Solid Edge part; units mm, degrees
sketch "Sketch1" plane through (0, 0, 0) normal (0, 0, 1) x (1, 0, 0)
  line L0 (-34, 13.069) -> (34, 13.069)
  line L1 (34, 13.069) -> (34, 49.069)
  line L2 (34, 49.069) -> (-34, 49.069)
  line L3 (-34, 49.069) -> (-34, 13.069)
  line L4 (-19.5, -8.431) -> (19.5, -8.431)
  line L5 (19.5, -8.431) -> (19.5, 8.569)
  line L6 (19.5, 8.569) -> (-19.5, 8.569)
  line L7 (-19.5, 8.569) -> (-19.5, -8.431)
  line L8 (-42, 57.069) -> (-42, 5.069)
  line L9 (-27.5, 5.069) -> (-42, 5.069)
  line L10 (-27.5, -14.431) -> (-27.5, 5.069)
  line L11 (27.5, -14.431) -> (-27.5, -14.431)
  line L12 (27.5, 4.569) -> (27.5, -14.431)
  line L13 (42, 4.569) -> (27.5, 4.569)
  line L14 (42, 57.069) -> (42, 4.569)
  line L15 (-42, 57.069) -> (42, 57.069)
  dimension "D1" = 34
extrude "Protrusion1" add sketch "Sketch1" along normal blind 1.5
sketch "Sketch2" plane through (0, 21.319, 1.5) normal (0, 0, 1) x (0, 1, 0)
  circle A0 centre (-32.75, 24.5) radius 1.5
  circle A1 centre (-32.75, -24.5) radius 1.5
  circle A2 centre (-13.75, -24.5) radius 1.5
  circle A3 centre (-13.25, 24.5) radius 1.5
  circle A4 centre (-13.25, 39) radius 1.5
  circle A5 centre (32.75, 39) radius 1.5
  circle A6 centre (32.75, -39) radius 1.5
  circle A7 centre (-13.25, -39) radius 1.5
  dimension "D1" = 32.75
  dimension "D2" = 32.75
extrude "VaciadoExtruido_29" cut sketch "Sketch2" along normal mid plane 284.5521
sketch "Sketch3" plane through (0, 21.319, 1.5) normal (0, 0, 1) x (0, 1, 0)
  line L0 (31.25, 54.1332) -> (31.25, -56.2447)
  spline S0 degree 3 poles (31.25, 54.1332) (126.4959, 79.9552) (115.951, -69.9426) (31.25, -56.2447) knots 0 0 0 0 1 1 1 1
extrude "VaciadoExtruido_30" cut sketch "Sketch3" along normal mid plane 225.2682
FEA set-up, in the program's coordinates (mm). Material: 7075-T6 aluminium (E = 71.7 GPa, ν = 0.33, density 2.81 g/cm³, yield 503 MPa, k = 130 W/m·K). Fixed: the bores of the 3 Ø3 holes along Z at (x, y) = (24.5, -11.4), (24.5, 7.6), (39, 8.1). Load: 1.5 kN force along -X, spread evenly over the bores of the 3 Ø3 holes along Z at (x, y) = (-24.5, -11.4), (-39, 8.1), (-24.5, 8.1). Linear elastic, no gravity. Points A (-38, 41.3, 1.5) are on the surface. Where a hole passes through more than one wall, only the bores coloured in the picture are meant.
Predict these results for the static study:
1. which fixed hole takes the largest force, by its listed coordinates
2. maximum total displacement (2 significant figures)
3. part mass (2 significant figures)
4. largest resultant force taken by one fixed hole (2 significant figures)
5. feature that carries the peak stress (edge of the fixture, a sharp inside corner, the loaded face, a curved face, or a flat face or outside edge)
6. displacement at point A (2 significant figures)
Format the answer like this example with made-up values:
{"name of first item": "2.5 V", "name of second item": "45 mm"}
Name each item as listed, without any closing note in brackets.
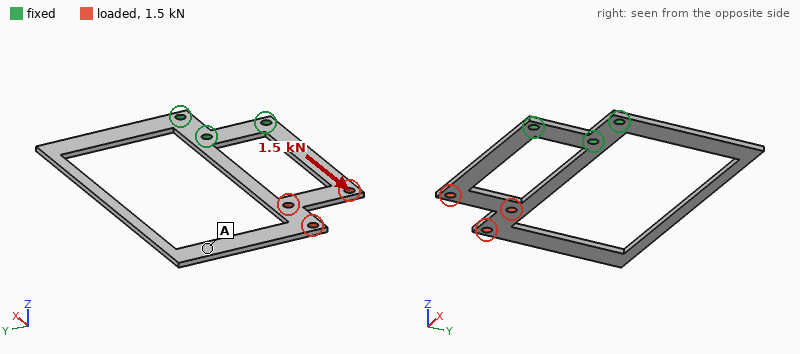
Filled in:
{"which fixed hole takes the largest force, by its listed coordinates": "(24.5, 7.6)", "maximum total displacement": "0.12 mm", "part mass": "8.1 g", "largest resultant force taken by one fixed hole": "770 N", "feature that carries the peak stress": "the loaded face", "displacement at point A": "0.046 mm"}
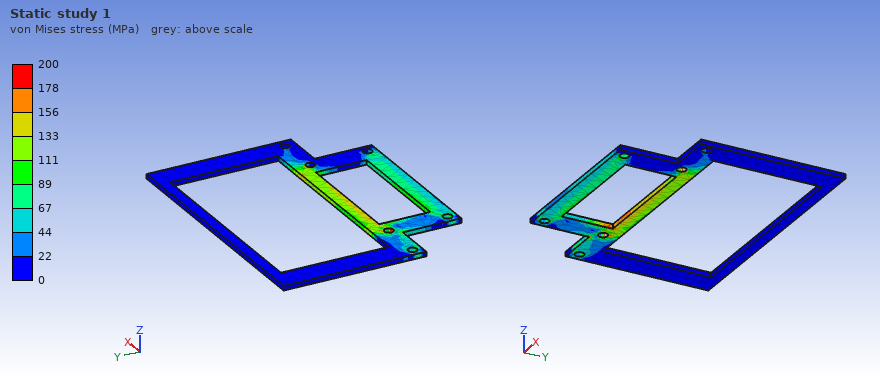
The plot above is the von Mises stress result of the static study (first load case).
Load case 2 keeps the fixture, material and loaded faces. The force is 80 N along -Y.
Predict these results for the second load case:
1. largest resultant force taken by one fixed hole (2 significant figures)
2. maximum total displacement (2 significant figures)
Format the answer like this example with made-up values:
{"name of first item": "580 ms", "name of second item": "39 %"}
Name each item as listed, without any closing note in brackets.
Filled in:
{"largest resultant force taken by one fixed hole": "150 N", "maximum total displacement": "0.28 mm"}
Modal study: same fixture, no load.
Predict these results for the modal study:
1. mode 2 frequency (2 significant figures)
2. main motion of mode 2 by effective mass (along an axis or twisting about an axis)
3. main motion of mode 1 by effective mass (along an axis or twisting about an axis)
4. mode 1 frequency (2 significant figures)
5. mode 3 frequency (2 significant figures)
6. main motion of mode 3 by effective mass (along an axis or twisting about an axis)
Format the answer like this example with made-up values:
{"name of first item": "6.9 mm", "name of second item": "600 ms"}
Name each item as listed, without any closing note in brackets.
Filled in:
{"mode 2 frequency": "390 Hz", "main motion of mode 2 by effective mass": "twisting about X", "main motion of mode 1 by effective mass": "along Z", "mode 1 frequency": "160 Hz", "mode 3 frequency": "620 Hz", "main motion of mode 3 by effective mass": "along Z"}
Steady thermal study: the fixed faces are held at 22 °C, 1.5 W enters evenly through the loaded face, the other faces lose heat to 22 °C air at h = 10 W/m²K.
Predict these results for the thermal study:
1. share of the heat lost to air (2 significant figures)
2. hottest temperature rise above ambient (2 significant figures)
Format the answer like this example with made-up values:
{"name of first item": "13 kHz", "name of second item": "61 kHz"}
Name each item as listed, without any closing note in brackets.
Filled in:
{"share of the heat lost to air": "33 %", "hottest temperature rise above ambient": "24 K"}
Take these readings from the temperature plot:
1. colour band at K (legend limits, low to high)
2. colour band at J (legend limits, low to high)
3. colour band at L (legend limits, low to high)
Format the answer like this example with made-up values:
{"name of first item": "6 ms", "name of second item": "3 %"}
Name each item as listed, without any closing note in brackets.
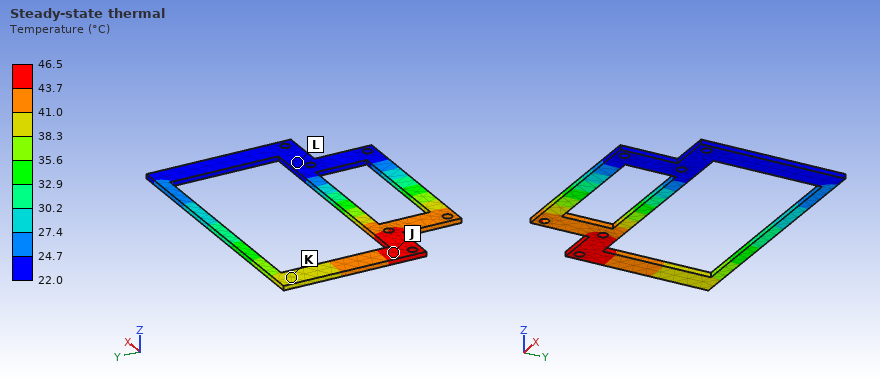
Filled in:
{"colour band at K": "38.3 to 41.0 °C", "colour band at J": "43.7 to 46.5 °C", "colour band at L": "22.0 to 24.7 °C"}
